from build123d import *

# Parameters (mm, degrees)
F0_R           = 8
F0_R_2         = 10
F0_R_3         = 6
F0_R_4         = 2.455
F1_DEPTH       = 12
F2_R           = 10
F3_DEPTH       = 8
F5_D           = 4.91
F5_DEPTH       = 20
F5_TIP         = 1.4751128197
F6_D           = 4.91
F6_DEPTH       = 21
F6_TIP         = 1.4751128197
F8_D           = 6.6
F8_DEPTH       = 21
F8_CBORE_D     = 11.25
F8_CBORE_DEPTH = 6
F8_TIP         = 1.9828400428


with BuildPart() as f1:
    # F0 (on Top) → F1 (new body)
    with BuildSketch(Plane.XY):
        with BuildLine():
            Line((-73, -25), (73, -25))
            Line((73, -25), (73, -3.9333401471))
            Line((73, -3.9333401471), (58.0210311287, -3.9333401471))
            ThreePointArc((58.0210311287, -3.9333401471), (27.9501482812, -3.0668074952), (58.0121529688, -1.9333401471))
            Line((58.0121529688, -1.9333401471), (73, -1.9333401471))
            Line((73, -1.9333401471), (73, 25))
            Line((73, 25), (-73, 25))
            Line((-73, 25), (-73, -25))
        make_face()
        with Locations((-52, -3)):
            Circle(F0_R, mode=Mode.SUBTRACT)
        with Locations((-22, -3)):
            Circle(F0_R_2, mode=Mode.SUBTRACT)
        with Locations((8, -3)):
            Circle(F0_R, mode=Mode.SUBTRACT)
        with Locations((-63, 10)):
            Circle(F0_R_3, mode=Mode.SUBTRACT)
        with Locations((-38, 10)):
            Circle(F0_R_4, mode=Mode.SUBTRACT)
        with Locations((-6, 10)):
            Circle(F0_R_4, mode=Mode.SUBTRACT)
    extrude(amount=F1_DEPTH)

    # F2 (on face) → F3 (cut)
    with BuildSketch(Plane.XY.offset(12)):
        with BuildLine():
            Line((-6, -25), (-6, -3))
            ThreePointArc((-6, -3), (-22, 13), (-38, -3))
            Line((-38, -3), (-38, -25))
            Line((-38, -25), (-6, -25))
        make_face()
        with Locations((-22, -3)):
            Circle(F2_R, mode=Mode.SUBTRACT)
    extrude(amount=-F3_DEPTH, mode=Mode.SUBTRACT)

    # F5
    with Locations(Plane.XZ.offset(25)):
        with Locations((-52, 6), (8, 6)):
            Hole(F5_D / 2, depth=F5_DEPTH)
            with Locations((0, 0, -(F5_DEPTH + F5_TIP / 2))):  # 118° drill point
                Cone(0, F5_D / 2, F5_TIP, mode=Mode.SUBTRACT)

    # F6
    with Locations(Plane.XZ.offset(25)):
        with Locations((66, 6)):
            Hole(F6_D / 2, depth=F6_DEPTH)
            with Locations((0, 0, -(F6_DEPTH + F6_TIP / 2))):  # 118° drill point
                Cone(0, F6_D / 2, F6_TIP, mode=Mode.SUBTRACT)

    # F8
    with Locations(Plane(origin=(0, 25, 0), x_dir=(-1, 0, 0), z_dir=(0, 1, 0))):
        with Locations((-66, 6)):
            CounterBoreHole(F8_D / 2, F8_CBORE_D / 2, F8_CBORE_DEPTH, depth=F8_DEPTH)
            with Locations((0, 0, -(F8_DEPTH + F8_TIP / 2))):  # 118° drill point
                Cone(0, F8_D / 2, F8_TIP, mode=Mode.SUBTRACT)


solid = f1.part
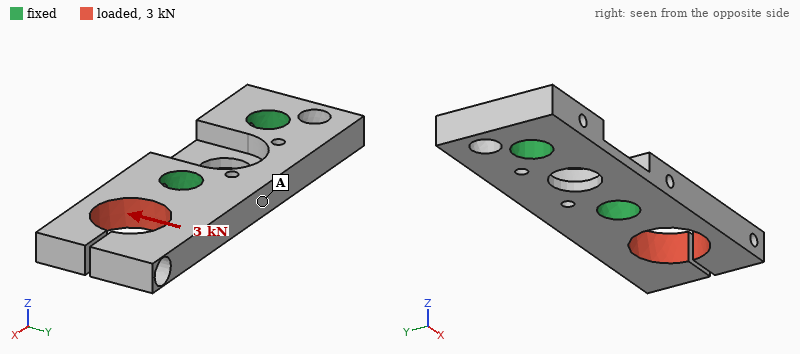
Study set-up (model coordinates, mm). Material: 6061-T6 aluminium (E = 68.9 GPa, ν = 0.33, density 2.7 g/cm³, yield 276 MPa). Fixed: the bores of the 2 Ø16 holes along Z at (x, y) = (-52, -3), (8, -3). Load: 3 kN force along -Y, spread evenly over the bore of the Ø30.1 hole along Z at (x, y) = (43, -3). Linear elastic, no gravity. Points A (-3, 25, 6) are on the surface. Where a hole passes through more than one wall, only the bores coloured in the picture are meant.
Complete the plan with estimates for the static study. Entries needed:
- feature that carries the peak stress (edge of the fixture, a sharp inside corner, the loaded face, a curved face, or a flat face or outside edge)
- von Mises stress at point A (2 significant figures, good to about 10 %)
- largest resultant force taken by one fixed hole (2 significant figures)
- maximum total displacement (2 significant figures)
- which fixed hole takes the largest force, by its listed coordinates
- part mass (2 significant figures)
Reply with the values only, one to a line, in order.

the loaded face
12 MPa
3.5 kN
0.28 mm
(8, -3)
160 g
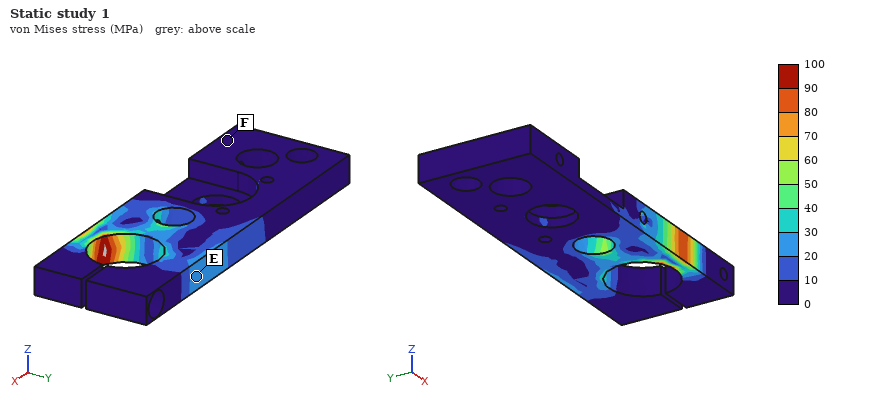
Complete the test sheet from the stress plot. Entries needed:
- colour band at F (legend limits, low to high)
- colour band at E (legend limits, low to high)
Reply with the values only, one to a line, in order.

0 to 10 MPa
20 to 30 MPa
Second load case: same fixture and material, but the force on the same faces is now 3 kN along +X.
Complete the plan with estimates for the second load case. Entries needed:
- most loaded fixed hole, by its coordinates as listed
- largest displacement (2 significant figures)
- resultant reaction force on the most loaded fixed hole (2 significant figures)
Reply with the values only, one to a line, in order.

(8, -3)
0.16 mm
2.8 kN
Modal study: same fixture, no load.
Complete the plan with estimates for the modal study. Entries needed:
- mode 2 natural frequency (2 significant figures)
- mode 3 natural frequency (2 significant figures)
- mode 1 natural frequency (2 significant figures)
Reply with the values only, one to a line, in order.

2300 Hz
2500 Hz
2100 Hz
